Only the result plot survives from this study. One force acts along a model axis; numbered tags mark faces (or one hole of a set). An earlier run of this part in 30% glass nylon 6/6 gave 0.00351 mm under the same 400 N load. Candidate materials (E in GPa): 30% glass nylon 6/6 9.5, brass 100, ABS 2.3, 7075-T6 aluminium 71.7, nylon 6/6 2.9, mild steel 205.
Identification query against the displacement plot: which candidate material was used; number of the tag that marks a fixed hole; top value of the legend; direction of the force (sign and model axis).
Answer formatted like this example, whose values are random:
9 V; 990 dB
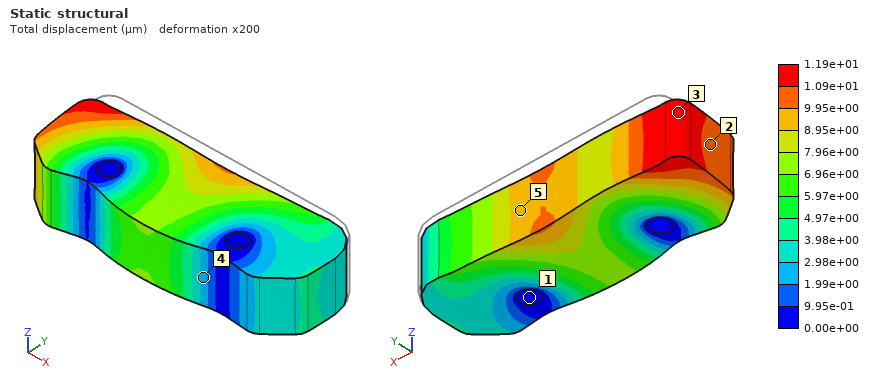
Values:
nylon 6/6; 1; 1.19e+01 µm; -Y
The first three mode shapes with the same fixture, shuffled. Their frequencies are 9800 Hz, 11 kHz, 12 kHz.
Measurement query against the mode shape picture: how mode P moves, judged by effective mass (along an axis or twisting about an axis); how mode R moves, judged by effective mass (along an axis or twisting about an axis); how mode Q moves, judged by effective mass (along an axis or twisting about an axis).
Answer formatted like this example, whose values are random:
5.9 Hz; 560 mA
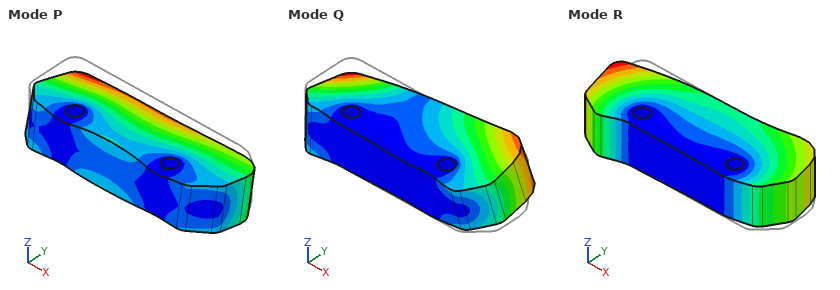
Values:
along Z; along X; twisting about Y
